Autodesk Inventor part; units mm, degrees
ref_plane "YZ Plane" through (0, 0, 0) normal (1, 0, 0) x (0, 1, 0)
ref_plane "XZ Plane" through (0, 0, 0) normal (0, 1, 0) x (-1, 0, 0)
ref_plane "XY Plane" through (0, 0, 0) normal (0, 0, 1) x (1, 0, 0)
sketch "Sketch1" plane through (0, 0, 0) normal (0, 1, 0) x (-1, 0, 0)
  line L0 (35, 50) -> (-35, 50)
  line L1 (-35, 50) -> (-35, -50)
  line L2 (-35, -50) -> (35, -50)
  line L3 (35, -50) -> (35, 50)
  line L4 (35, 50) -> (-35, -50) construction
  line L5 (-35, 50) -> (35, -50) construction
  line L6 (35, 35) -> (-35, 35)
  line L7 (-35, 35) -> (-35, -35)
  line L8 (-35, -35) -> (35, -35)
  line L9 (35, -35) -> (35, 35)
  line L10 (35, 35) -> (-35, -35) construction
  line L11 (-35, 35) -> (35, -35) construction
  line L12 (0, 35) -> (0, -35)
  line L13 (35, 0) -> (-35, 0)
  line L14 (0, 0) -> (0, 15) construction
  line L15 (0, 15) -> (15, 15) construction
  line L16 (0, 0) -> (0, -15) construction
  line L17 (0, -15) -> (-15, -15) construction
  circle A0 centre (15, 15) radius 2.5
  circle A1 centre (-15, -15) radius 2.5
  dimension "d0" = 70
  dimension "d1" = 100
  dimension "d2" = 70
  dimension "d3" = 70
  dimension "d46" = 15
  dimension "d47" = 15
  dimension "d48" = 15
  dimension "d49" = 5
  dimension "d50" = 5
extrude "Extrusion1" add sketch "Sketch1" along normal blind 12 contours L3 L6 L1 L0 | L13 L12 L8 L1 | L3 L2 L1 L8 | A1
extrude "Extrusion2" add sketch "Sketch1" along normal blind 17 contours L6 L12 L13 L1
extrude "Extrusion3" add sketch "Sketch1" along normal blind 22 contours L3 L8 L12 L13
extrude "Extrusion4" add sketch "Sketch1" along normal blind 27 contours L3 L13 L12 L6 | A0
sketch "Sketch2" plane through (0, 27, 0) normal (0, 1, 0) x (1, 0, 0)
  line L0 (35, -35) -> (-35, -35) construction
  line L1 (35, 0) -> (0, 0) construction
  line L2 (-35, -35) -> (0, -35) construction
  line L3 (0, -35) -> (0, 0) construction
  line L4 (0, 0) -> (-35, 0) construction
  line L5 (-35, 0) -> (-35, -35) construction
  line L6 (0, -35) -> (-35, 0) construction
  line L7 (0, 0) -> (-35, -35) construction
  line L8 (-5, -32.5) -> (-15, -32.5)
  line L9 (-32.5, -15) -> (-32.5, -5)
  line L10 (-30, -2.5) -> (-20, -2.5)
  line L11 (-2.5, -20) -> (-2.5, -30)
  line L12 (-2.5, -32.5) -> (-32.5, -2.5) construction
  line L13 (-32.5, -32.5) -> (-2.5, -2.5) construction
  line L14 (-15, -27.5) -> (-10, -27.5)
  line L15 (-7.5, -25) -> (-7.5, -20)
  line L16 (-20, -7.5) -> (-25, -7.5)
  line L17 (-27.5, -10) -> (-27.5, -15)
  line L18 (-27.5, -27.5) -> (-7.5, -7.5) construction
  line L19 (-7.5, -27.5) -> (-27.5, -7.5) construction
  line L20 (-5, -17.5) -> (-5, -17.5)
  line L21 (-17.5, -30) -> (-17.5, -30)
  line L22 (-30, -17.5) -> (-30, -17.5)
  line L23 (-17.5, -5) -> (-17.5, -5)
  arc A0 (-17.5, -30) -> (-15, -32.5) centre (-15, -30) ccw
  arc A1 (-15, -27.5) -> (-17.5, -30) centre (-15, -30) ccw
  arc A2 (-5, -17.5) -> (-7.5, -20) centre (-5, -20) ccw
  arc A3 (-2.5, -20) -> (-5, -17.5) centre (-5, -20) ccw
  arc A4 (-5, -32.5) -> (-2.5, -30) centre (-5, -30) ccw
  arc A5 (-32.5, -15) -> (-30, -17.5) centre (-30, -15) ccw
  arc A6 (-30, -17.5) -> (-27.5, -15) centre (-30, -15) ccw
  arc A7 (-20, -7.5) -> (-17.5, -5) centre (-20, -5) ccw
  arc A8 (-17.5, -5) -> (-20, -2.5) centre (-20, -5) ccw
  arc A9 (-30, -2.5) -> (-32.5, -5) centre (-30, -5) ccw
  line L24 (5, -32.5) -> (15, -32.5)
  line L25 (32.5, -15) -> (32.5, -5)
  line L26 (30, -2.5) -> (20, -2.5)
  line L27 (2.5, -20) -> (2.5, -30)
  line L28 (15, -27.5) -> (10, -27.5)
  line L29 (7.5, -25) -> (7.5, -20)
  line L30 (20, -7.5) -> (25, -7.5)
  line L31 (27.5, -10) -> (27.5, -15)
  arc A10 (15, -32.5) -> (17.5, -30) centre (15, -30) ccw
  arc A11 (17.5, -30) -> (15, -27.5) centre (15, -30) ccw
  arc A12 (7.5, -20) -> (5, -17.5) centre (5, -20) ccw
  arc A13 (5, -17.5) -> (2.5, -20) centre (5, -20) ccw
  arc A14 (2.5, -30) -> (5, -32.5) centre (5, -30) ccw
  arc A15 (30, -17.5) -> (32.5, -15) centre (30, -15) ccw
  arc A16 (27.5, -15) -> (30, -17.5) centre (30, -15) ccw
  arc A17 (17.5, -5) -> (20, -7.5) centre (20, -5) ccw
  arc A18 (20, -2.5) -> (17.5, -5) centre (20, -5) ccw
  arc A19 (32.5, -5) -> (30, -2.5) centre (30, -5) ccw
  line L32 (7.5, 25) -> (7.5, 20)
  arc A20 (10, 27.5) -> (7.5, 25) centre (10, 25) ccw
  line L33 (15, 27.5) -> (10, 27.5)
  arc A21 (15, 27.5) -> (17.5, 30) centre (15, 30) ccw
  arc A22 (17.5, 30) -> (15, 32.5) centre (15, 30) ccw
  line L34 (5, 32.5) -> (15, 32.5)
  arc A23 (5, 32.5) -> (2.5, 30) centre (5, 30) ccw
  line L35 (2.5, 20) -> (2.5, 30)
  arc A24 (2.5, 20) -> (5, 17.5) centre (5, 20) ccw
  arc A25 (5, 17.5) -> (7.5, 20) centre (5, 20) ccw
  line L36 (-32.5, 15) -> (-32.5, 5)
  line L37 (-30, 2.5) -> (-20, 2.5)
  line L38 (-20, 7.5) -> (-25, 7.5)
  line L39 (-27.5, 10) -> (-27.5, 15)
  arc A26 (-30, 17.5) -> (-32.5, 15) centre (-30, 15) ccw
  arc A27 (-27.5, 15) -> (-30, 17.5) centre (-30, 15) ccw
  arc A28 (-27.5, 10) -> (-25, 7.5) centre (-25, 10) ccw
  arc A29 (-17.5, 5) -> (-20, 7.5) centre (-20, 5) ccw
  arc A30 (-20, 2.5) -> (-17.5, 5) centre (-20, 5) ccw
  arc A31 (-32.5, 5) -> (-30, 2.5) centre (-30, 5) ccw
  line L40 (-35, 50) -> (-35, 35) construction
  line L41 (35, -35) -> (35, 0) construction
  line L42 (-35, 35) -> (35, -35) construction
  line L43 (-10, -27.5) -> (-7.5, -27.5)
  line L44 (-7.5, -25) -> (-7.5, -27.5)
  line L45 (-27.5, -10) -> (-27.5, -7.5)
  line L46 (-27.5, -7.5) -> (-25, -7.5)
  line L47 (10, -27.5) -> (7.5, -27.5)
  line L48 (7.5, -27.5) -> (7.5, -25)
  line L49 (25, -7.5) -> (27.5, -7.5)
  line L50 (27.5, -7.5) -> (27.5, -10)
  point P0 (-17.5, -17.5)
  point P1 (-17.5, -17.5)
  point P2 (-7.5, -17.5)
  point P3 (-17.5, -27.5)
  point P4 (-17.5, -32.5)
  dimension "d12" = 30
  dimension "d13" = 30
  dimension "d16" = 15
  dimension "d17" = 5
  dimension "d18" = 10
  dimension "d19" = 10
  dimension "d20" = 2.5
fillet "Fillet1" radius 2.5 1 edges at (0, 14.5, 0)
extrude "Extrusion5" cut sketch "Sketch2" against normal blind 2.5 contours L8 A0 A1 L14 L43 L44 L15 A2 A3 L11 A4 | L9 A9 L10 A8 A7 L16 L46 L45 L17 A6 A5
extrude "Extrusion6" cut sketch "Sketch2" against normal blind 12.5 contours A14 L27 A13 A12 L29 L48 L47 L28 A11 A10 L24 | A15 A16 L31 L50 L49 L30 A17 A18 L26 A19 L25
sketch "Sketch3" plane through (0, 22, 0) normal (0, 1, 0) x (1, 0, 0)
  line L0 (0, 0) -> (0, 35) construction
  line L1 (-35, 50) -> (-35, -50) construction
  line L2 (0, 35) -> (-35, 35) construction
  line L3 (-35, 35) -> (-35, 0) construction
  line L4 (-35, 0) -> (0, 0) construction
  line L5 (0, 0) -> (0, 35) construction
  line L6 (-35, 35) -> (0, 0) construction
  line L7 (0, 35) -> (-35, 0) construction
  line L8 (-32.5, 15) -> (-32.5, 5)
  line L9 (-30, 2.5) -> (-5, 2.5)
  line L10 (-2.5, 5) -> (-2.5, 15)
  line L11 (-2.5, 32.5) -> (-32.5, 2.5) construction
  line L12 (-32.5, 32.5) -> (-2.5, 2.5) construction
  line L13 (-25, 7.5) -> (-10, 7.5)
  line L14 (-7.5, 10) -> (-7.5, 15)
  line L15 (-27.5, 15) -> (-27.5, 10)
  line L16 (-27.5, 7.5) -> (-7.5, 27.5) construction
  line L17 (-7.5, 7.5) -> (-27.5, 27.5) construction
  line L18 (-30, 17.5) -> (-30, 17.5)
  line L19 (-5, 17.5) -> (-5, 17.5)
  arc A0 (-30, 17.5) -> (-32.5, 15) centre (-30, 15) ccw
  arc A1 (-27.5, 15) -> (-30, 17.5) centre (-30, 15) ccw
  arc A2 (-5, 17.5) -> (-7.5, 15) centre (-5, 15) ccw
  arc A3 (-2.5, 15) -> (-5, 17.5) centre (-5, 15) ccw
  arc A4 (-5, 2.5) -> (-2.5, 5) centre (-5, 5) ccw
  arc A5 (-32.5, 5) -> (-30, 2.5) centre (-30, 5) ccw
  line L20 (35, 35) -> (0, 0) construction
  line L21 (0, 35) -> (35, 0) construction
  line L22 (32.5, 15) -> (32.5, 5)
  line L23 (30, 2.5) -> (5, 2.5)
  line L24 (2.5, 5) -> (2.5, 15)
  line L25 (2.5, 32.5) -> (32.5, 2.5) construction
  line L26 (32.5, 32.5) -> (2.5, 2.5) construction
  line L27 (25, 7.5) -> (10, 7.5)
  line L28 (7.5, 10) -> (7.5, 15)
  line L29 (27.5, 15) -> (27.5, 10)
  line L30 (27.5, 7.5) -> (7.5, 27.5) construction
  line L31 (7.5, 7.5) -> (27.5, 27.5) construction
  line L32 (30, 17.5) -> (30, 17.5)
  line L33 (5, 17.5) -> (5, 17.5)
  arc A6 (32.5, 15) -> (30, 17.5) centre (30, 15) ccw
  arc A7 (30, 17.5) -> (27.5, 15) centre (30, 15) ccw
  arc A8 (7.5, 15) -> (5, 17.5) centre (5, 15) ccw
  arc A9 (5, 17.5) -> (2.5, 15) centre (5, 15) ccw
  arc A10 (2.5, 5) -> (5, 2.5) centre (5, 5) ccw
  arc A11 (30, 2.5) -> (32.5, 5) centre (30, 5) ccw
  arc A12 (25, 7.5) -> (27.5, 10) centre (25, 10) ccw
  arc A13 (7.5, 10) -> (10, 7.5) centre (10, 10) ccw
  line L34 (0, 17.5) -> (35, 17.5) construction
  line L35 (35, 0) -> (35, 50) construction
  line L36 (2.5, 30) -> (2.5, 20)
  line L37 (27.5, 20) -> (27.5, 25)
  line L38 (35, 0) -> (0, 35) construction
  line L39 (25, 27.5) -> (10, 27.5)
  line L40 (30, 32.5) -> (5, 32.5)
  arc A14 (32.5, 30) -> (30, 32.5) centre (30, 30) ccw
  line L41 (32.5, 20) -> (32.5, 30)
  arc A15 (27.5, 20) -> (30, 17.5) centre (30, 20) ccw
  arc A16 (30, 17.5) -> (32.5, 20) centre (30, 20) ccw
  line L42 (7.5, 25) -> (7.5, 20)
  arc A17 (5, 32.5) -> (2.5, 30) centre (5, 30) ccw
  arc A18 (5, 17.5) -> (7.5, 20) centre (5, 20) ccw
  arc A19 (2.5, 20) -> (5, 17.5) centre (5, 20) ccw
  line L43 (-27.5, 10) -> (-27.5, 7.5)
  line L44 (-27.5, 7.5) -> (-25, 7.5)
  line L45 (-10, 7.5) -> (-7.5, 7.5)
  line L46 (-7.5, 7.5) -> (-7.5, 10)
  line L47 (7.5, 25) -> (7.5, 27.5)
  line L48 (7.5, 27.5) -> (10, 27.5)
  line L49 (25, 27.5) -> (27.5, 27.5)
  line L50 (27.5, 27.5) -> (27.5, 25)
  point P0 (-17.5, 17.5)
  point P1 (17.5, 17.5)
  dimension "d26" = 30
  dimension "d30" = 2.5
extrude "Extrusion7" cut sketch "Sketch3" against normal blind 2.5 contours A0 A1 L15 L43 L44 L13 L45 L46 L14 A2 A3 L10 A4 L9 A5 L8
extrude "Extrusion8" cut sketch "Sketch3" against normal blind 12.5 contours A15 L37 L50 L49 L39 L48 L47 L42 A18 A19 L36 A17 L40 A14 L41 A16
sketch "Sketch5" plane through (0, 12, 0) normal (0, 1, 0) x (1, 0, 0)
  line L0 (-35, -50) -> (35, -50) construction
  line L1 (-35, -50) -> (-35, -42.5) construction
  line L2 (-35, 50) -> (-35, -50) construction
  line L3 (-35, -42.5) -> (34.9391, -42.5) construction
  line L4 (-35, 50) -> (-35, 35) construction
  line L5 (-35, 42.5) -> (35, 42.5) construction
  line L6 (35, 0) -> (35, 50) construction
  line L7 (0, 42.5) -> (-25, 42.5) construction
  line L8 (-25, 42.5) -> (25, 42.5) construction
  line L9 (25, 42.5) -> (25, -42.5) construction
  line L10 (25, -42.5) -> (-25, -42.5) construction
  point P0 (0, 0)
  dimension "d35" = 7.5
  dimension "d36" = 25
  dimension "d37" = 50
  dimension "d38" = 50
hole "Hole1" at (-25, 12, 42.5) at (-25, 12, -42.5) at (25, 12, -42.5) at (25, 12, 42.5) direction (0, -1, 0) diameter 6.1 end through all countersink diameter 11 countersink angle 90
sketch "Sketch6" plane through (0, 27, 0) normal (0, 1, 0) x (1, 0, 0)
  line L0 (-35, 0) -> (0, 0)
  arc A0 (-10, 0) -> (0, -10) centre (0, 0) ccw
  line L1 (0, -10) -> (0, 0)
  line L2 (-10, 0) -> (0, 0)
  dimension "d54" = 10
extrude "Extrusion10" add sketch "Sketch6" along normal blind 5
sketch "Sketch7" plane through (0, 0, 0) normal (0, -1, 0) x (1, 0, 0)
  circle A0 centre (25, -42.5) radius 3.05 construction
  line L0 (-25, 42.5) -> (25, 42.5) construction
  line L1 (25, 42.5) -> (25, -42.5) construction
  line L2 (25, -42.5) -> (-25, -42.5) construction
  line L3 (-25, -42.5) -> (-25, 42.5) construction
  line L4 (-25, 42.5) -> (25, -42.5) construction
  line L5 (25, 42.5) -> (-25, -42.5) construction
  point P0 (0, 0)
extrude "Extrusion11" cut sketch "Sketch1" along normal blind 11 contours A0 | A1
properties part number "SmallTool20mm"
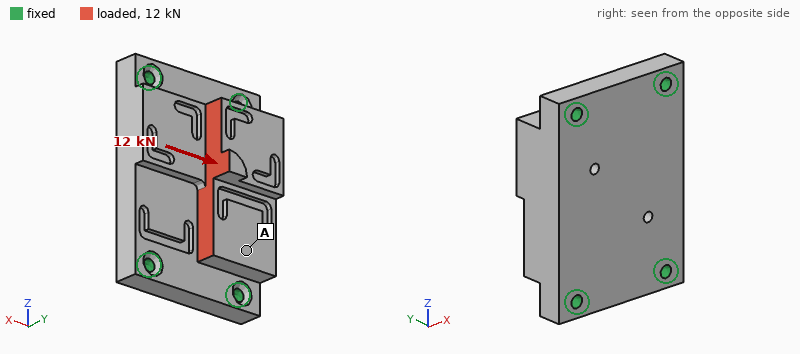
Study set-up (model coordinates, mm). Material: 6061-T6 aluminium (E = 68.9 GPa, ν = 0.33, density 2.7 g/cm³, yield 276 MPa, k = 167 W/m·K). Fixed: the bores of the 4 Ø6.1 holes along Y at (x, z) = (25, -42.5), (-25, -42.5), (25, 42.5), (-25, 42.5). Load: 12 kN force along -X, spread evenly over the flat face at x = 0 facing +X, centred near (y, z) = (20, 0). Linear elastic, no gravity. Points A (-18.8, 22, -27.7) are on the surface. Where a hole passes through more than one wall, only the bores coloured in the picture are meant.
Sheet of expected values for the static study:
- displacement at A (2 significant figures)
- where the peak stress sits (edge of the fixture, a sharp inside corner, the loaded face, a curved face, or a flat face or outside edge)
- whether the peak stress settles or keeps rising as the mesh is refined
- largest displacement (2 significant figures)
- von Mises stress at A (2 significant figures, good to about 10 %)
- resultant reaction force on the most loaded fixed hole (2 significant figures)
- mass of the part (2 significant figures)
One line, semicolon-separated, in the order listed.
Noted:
16 µm; edge of the fixture; keeps rising; 40 µm; 11 MPa; 4.5 kN; 310 g
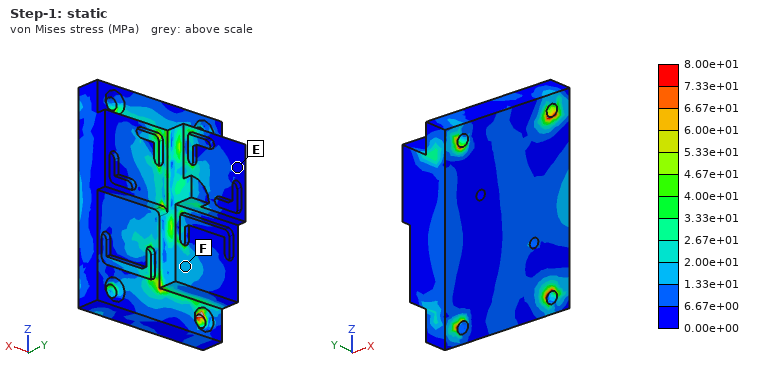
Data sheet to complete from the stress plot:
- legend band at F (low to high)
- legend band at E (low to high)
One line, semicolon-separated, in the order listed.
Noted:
1.33e+01 to 2.00e+01 MPa; 0.00e+00 to 6.67e+00 MPa
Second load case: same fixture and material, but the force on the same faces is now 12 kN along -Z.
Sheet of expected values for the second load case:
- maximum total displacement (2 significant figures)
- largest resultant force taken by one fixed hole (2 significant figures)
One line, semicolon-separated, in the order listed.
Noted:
28 µm; 4.6 kN
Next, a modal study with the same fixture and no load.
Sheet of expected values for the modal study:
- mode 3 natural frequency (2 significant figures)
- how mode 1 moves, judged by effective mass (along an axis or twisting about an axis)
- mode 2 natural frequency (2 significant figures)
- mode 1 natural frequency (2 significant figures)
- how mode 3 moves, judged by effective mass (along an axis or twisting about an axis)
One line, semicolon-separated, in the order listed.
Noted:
12 kHz; along Y; 9100 Hz; 6800 Hz; along X
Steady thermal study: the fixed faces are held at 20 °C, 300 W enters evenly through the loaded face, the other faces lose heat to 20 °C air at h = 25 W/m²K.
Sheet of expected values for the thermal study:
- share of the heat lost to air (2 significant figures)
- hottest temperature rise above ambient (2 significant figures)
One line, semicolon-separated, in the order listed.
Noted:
3.8 %; 69 K
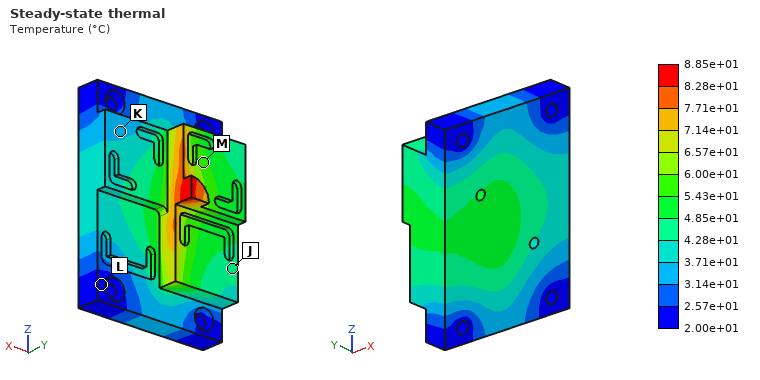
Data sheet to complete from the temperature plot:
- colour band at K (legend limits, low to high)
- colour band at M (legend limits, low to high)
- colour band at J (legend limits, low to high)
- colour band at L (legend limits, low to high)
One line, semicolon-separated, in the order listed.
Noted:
3.14e+01 to 3.71e+01 °C; 5.43e+01 to 6.00e+01 °C; 4.28e+01 to 4.85e+01 °C; 2.00e+01 to 2.57e+01 °C
